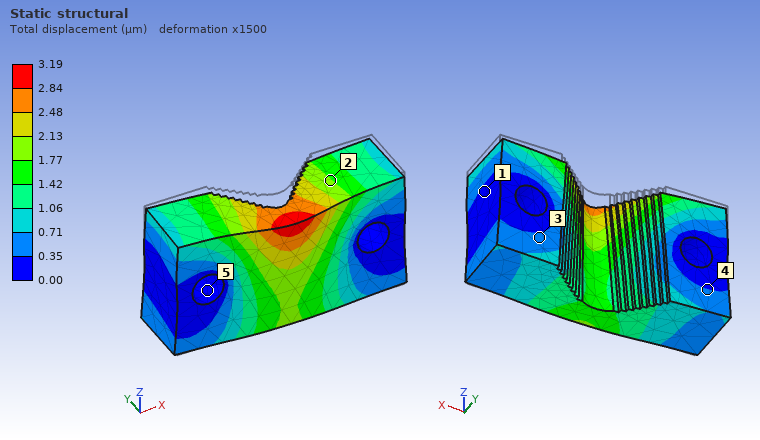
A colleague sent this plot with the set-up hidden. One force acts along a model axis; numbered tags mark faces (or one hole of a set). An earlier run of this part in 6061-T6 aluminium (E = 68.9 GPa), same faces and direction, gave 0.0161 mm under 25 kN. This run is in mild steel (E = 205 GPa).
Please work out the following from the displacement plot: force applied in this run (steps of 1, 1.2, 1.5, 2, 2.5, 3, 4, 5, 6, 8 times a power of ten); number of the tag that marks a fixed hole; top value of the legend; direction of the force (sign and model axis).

15 kN
5
3.19 µm
-Z
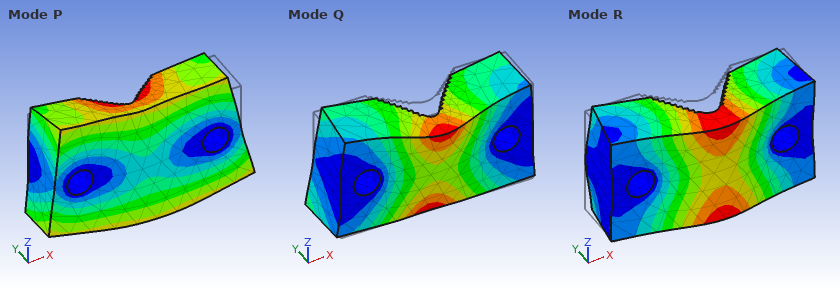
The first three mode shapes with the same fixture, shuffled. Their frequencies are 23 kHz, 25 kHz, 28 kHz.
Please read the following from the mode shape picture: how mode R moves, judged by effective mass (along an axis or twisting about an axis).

along Y
